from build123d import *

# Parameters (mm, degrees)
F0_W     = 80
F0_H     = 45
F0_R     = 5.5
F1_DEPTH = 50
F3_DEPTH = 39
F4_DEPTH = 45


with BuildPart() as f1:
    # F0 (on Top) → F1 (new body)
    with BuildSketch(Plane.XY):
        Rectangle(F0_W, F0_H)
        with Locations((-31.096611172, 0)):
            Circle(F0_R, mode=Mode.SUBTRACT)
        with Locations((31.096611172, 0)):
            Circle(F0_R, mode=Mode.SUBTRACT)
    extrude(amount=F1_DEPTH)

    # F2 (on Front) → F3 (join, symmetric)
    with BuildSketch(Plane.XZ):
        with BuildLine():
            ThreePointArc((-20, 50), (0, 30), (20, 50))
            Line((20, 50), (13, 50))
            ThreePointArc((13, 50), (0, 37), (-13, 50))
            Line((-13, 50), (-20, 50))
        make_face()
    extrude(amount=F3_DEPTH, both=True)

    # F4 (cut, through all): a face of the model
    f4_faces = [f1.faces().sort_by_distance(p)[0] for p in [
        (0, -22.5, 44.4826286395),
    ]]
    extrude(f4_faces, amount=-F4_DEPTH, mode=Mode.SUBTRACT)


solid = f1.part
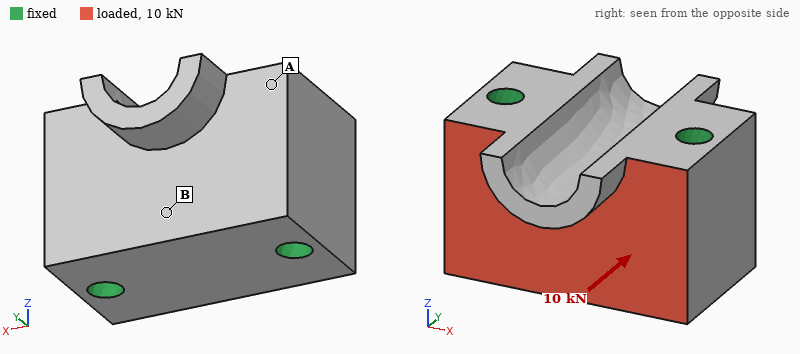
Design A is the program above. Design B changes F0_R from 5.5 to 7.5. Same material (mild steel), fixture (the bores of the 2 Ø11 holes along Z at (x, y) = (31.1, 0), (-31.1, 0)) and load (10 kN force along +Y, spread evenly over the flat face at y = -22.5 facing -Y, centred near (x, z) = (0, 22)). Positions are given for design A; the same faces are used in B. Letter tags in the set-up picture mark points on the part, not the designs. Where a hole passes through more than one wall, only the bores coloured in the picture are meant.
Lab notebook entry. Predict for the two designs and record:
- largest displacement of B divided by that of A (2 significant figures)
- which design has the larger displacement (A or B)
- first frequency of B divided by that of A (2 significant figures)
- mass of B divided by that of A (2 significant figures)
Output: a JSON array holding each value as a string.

["0.86", "A", "1.0", "0.95"]
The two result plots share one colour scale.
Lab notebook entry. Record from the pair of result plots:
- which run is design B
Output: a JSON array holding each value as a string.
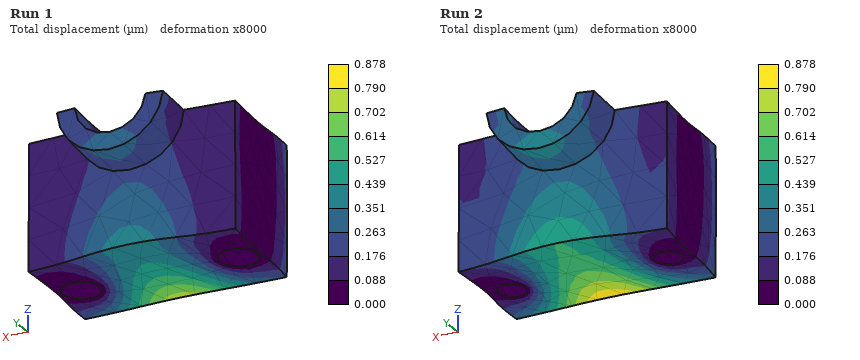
["Run 1"]
